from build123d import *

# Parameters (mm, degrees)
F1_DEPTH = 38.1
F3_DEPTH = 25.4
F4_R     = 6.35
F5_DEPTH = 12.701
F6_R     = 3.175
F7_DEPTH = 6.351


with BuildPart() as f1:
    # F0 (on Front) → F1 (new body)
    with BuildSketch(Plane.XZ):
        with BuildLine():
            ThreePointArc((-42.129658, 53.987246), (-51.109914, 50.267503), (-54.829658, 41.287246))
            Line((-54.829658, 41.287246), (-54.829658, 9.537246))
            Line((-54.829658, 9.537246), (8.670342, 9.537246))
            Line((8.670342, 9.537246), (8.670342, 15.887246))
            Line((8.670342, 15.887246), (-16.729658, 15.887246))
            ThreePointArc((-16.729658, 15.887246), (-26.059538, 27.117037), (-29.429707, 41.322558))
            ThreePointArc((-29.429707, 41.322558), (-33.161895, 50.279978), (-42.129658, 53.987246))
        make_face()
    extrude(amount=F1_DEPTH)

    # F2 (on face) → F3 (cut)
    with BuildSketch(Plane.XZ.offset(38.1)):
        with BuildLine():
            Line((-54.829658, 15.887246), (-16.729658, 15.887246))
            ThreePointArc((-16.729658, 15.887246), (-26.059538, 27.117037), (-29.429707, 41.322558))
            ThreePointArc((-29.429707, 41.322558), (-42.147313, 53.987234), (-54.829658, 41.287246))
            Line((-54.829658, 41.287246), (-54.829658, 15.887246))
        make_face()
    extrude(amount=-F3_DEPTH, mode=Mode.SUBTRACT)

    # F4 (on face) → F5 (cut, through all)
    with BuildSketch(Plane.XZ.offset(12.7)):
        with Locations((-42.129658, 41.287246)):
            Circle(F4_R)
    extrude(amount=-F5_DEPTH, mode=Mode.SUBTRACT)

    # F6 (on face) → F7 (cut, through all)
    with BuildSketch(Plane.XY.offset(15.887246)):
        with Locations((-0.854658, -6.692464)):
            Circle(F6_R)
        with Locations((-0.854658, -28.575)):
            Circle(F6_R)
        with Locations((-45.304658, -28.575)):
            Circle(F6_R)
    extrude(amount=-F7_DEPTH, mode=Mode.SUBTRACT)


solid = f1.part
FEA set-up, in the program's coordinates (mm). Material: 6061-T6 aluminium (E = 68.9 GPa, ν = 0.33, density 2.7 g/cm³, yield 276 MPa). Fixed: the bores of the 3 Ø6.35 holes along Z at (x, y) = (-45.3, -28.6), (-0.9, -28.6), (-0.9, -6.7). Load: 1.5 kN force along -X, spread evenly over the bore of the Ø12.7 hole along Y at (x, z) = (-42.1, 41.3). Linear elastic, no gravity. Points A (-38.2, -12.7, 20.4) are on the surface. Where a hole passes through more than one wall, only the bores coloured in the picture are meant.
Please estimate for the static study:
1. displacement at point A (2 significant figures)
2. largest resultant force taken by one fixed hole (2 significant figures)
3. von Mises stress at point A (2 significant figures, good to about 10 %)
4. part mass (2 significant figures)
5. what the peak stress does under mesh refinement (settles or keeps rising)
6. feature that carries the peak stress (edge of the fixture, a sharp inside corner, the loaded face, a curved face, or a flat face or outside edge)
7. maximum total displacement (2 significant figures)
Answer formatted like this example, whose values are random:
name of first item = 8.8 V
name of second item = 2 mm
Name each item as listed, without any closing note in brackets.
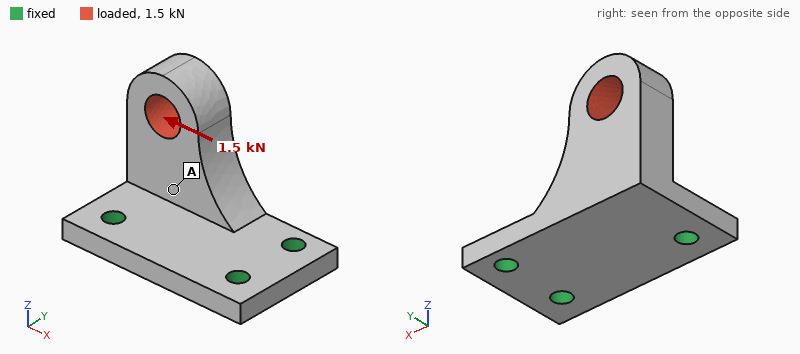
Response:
displacement at point A = 0.031 mm
largest resultant force taken by one fixed hole = 1.1 kN
von Mises stress at point A = 17 MPa
part mass = 70 g
what the peak stress does under mesh refinement = keeps rising
feature that carries the peak stress = edge of the fixture
maximum total displacement = 0.14 mm
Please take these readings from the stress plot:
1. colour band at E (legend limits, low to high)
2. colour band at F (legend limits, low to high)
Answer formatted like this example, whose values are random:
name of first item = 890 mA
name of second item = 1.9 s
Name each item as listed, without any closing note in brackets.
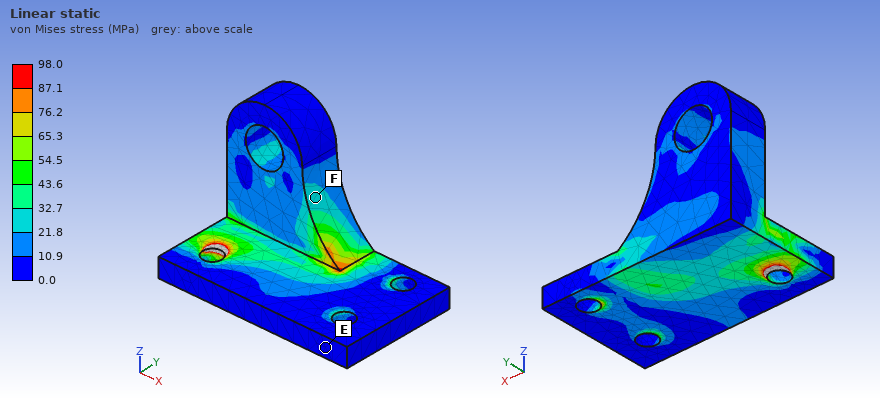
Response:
colour band at E = 0.0 to 10.9 MPa
colour band at F = 21.8 to 32.7 MPa
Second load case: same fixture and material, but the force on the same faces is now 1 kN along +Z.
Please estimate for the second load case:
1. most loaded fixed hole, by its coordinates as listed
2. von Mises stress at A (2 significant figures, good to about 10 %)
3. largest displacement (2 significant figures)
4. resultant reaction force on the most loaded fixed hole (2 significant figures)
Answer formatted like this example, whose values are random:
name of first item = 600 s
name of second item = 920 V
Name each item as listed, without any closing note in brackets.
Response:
most loaded fixed hole, by its coordinates as listed = (-45.3, -28.6)
von Mises stress at A = 9.3 MPa
largest displacement = 0.11 mm
resultant reaction force on the most loaded fixed hole = 810 N
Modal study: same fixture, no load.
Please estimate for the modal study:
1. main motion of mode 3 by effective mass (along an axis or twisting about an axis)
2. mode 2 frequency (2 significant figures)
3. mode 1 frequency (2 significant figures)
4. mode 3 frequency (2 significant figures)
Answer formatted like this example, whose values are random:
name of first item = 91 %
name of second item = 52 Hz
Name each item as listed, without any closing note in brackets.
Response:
main motion of mode 3 by effective mass = along Z
mode 2 frequency = 5600 Hz
mode 1 frequency = 2500 Hz
mode 3 frequency = 8200 Hz
